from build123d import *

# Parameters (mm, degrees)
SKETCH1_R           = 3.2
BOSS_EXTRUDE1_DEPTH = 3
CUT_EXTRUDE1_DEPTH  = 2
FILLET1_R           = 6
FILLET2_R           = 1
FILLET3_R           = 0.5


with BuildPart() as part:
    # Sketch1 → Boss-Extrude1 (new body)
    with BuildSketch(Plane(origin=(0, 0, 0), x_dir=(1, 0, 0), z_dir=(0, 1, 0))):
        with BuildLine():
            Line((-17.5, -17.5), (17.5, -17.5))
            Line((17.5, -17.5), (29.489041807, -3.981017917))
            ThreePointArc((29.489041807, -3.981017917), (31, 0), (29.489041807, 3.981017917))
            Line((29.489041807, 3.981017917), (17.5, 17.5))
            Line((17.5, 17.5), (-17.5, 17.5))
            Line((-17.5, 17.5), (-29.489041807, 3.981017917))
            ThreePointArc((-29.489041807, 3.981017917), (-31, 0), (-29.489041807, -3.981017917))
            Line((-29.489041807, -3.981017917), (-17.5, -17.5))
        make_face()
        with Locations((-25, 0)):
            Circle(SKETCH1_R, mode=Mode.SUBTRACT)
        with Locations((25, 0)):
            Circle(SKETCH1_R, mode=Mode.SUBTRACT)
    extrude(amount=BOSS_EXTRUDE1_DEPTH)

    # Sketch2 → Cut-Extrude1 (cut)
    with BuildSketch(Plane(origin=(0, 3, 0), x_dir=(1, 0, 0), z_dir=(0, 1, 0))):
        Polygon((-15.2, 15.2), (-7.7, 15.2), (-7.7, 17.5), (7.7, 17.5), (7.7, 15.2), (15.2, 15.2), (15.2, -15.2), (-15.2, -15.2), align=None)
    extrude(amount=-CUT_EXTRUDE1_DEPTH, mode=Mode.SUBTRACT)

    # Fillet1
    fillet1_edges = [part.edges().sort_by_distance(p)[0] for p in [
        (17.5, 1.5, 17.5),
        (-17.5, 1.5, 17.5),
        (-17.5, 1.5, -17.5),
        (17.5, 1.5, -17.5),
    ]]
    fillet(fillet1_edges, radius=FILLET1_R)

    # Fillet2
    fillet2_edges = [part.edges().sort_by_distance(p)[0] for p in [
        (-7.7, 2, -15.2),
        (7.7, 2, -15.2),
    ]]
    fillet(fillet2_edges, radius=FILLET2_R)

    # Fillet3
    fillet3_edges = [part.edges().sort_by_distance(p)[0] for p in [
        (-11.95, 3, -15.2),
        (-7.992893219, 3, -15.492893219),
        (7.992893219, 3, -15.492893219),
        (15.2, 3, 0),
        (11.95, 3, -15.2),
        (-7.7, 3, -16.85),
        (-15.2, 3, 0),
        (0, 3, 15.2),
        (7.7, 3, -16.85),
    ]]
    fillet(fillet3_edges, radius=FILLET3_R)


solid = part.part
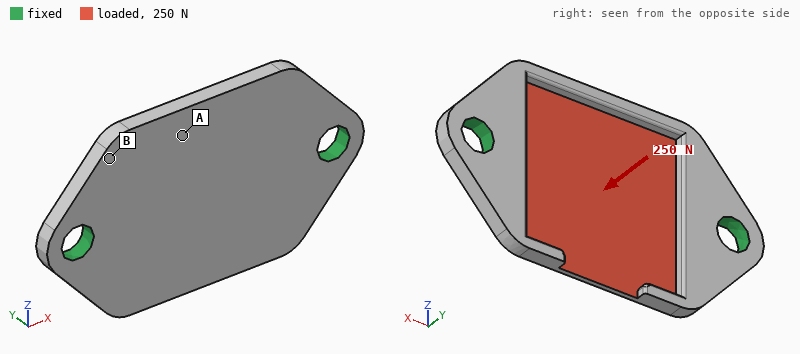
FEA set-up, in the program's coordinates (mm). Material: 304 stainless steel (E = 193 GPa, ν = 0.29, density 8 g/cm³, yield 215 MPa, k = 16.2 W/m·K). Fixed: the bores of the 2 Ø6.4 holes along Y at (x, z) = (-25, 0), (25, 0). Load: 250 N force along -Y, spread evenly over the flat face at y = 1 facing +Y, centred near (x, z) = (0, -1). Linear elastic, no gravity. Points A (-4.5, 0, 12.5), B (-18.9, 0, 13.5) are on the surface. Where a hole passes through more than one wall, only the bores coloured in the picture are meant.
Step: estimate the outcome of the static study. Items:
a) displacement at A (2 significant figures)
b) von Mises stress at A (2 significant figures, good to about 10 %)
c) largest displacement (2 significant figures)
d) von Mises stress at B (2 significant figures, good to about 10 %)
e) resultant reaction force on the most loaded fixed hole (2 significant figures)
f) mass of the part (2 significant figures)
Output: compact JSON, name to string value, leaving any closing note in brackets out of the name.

{"displacement at A": "21 µm", "von Mises stress at A": "31 MPa", "largest displacement": "39 µm", "von Mises stress at B": "11 MPa", "resultant reaction force on the most loaded fixed hole": "230 N", "mass of the part": "25 g"}
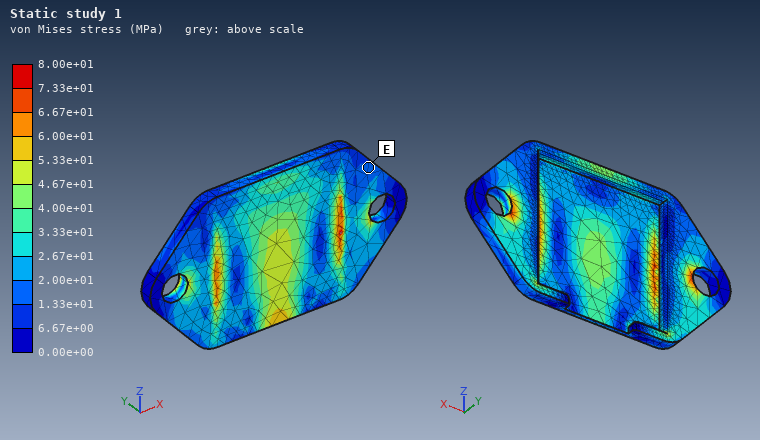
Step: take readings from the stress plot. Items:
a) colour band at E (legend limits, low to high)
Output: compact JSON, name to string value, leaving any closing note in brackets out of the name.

{"colour band at E": "1.33e+01 to 2.00e+01 MPa"}
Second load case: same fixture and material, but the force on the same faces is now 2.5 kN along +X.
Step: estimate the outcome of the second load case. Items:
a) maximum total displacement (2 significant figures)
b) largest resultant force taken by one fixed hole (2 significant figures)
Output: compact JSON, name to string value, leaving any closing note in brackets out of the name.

{"maximum total displacement": "11 µm", "largest resultant force taken by one fixed hole": "1.3 kN"}
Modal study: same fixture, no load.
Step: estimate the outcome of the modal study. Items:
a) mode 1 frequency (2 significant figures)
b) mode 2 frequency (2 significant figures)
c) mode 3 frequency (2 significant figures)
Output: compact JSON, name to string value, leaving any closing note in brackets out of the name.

{"mode 1 frequency": "5000 Hz", "mode 2 frequency": "5200 Hz", "mode 3 frequency": "8400 Hz"}
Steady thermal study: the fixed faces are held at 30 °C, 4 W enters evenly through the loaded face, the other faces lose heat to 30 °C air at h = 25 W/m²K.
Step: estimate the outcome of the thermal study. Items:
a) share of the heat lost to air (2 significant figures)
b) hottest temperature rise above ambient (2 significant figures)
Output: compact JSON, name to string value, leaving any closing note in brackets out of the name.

{"share of the heat lost to air": "30 %", "hottest temperature rise above ambient": "35 K"}
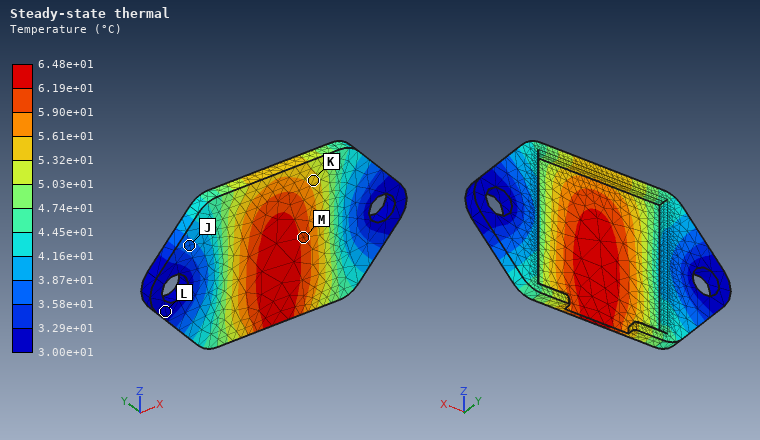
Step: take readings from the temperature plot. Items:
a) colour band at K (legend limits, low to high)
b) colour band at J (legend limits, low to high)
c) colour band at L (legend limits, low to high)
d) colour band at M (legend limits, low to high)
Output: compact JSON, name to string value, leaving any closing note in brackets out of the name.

{"colour band at K": "5.32e+01 to 5.61e+01 °C", "colour band at J": "3.58e+01 to 3.87e+01 °C", "colour band at L": "3.00e+01 to 3.29e+01 °C", "colour band at M": "5.90e+01 to 6.19e+01 °C"}
